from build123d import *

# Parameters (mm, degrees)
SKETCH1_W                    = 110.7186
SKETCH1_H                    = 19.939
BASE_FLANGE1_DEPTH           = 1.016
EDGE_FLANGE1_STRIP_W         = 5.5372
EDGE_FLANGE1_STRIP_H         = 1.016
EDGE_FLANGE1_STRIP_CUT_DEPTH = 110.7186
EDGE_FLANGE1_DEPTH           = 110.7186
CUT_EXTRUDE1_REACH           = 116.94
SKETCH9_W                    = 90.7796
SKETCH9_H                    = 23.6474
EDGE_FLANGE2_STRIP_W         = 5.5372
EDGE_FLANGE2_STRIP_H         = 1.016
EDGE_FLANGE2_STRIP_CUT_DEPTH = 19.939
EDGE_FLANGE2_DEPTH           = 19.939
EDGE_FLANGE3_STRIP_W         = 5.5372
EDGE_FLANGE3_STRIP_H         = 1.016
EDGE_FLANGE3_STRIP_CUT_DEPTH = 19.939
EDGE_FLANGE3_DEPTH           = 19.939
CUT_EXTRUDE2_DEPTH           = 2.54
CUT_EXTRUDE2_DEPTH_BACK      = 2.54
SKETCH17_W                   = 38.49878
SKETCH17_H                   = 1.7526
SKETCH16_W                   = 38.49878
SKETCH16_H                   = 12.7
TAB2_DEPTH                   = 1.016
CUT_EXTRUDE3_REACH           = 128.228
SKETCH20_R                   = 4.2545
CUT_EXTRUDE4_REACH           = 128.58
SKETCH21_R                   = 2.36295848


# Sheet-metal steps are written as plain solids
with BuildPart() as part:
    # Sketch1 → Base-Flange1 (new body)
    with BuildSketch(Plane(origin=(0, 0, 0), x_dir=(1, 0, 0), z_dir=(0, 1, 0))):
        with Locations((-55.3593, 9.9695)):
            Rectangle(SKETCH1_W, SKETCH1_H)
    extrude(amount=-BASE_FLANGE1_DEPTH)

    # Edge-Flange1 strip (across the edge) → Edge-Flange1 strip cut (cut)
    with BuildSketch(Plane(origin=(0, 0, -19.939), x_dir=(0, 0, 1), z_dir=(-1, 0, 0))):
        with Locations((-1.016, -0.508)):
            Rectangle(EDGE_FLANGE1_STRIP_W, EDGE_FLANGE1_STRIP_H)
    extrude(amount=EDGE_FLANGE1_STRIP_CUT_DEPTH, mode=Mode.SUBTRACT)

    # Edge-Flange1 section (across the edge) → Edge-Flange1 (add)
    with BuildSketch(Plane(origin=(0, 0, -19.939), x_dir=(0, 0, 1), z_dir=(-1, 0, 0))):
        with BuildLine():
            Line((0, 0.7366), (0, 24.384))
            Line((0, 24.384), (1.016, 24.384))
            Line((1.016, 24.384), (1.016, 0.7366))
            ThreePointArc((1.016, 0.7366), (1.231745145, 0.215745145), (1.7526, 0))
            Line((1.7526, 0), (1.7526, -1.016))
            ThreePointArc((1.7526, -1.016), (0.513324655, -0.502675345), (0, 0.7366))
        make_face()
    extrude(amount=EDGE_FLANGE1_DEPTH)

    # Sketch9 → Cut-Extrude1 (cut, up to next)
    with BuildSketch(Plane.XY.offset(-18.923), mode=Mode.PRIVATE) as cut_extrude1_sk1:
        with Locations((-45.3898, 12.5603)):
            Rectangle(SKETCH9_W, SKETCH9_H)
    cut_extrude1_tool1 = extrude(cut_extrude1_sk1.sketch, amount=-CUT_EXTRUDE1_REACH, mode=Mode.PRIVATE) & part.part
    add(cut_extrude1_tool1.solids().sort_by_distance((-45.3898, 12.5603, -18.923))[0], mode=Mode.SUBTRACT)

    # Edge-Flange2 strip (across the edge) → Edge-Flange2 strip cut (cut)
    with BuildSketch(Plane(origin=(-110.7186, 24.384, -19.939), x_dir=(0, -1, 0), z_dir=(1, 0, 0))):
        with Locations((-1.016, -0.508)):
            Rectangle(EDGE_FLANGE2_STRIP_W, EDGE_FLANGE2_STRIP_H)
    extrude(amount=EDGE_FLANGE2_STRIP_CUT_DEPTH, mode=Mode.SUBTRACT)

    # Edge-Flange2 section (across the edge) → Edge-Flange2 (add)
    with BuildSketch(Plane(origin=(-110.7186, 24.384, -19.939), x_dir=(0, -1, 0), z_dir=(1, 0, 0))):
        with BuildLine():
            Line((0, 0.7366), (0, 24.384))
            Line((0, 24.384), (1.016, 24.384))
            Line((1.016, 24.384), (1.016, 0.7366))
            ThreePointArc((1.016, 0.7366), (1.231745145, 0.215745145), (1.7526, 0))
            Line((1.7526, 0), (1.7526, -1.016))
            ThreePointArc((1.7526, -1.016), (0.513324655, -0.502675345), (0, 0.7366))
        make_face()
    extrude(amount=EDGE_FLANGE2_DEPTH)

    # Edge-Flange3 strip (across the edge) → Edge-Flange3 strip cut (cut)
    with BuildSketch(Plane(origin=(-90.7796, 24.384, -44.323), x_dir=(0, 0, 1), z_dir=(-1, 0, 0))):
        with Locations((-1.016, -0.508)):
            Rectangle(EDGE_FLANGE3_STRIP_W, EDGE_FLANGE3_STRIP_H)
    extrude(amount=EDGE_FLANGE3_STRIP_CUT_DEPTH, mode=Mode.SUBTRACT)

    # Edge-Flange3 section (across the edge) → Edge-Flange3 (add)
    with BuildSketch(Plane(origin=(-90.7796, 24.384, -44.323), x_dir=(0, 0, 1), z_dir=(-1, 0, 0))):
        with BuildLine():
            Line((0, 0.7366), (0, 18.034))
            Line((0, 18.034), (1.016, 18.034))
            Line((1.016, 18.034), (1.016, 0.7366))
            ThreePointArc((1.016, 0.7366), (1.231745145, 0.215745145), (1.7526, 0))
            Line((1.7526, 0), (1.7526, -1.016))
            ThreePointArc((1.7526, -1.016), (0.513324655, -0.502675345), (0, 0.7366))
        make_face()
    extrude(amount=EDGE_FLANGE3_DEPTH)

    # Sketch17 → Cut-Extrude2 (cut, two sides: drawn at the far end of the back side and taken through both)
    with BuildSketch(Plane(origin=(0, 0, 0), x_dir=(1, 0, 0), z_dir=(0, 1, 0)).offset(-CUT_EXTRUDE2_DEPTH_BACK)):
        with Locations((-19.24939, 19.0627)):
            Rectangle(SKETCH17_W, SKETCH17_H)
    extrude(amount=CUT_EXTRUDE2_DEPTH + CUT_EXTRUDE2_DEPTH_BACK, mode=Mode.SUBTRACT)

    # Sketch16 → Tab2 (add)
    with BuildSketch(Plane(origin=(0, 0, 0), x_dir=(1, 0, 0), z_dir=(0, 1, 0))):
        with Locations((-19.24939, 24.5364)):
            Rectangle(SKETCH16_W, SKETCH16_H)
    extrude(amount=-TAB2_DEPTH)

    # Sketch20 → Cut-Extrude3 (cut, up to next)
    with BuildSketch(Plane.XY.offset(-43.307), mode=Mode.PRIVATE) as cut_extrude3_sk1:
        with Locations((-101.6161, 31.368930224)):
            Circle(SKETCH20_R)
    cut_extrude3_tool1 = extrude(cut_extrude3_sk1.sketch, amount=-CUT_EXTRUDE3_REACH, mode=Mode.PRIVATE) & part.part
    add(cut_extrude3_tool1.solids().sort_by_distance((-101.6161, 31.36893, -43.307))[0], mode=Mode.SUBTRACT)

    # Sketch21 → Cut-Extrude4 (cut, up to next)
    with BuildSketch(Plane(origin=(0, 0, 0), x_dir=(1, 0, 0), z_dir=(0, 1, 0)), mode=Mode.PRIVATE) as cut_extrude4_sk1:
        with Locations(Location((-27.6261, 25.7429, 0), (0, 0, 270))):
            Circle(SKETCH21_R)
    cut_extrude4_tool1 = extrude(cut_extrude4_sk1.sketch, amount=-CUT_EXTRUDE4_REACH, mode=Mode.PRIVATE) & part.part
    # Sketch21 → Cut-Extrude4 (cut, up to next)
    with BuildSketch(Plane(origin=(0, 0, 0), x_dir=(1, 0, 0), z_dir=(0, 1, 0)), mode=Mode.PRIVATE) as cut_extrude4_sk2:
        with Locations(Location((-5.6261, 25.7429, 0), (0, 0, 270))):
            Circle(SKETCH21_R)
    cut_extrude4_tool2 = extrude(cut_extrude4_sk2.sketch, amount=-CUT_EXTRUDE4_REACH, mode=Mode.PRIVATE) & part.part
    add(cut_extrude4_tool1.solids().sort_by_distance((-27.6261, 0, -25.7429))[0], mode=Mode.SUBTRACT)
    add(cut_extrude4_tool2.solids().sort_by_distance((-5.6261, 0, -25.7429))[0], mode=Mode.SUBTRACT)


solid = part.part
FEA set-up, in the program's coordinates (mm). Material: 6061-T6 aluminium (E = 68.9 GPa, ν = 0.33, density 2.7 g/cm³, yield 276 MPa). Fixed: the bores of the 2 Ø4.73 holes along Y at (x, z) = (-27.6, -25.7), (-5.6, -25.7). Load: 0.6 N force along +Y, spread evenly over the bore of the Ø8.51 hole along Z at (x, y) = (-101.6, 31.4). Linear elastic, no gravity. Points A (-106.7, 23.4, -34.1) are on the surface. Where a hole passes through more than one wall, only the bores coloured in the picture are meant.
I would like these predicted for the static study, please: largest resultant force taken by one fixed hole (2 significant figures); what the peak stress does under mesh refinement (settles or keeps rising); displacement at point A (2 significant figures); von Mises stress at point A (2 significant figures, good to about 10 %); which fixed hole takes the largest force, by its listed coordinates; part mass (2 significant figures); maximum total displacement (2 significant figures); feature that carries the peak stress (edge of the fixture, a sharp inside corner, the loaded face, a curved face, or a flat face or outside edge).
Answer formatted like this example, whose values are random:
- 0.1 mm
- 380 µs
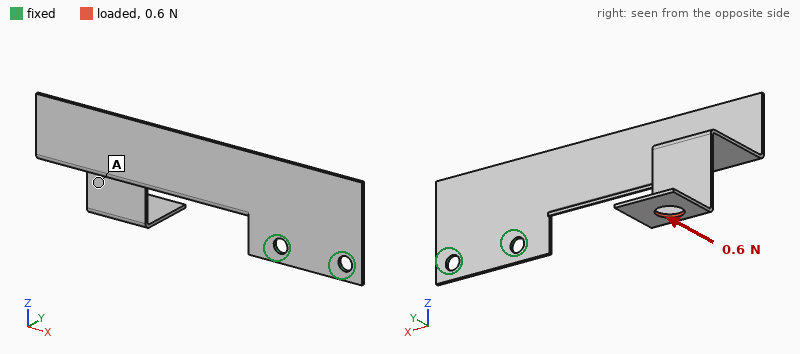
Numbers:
- 1.3 N
- keeps rising
- 0.92 mm
- 1.6 MPa
- (-27.6, -25.7)
- 11 g
- 1.2 mm
- a sharp inside corner
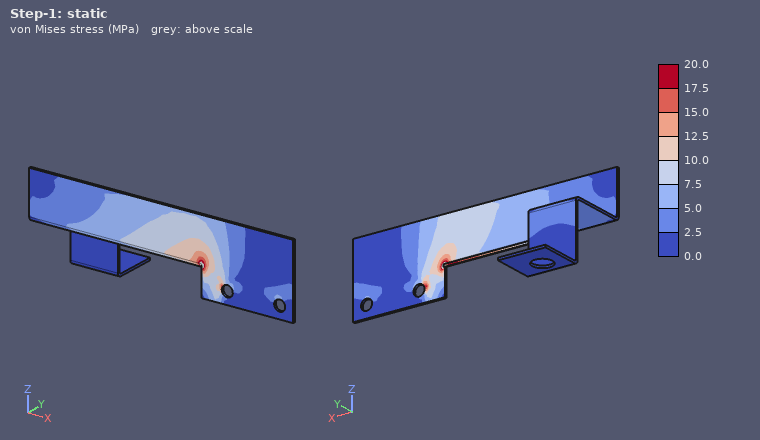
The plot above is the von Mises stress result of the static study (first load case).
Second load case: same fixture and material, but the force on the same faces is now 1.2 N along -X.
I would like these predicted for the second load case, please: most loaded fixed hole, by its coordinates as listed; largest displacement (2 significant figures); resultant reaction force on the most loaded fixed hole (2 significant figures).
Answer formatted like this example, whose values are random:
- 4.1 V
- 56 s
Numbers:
- (-27.6, -25.7)
- 1.2 mm
- 2.0 N
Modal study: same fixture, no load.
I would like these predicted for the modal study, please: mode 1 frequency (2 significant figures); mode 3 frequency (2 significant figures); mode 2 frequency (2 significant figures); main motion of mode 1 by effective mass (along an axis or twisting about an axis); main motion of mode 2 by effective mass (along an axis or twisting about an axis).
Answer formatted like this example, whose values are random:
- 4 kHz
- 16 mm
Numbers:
- 65 Hz
- 310 Hz
- 130 Hz
- along Y
- along Z
